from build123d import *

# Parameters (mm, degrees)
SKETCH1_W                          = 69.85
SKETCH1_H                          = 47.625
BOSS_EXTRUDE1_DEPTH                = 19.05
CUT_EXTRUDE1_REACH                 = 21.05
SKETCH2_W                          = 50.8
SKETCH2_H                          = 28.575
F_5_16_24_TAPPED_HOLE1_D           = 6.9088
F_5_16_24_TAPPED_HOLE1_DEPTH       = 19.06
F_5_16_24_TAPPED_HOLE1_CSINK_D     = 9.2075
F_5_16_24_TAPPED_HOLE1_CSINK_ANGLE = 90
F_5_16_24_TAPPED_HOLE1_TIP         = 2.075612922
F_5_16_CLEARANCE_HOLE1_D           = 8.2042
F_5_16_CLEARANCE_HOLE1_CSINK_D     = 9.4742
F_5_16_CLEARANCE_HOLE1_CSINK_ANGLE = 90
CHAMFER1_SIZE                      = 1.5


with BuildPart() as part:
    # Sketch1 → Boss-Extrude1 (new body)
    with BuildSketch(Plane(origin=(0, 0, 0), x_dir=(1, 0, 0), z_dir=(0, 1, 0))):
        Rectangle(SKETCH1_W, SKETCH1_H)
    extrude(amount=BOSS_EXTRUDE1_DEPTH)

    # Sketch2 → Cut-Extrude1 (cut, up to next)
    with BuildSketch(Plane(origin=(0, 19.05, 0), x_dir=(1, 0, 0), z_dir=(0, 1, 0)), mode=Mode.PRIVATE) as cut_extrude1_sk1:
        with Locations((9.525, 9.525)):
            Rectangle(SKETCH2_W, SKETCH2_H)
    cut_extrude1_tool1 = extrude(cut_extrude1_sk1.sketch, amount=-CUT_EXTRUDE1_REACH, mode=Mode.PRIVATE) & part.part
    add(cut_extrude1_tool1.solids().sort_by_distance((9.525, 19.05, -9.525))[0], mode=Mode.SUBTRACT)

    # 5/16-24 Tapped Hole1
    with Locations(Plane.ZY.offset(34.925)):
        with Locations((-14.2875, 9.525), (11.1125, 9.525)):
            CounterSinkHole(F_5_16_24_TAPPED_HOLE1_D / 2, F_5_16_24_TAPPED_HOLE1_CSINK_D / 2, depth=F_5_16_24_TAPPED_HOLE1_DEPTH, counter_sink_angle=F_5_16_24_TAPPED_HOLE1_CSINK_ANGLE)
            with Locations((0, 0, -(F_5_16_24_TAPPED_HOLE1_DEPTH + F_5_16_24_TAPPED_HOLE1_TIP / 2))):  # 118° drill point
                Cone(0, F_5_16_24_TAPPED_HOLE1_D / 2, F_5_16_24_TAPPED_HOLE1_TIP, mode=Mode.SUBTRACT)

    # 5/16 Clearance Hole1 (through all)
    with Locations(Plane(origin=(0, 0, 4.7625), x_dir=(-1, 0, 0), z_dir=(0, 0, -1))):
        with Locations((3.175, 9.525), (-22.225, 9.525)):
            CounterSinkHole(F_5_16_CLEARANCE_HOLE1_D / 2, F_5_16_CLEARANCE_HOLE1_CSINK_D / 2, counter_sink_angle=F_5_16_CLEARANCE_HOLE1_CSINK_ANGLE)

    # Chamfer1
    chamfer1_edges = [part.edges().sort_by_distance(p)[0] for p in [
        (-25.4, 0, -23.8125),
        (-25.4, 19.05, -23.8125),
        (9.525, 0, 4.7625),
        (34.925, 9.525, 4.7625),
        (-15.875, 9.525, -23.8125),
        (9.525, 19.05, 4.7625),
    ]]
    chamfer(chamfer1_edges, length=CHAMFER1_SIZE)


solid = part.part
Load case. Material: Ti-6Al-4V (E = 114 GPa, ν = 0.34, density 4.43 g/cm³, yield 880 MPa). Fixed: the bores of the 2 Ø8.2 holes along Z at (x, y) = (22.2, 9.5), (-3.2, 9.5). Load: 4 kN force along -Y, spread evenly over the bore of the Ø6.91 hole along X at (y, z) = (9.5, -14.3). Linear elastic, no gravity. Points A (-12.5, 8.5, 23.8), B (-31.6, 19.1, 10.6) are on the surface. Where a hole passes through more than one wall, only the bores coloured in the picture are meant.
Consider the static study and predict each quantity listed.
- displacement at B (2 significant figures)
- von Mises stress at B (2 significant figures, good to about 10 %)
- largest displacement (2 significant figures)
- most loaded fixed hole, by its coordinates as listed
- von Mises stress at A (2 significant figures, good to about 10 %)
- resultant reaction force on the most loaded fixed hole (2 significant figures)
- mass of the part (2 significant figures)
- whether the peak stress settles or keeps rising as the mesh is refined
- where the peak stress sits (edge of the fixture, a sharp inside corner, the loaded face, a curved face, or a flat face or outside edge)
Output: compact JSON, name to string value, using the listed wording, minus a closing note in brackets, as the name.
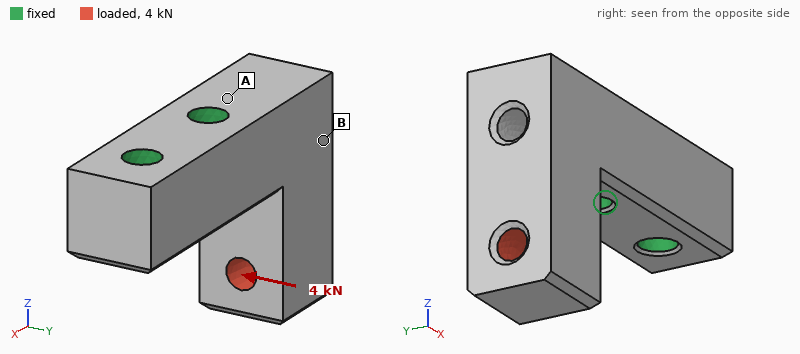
{"displacement at B": "0.041 mm", "von Mises stress at B": "34 MPa", "largest displacement": "0.15 mm", "most loaded fixed hole, by its coordinates as listed": "(-3.2, 9.5)", "von Mises stress at A": "76 MPa", "resultant reaction force on the most loaded fixed hole": "4.9 kN", "mass of the part": "140 g", "whether the peak stress settles or keeps rising as the mesh is refined": "keeps rising", "where the peak stress sits": "edge of the fixture"}
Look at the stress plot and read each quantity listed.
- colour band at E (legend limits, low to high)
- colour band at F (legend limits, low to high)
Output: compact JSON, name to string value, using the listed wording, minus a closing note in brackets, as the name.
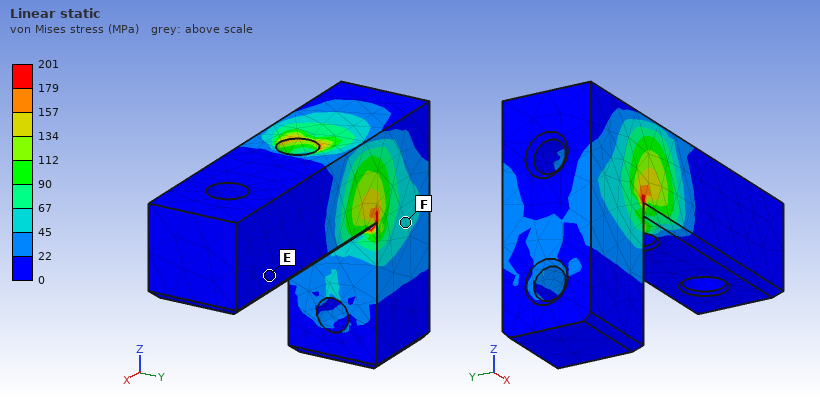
{"colour band at E": "0 to 22 MPa", "colour band at F": "45 to 67 MPa"}
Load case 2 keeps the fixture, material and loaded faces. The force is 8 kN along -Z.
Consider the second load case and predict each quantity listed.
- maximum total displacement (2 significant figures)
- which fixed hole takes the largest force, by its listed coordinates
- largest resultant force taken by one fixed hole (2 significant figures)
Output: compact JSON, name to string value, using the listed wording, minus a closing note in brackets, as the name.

{"maximum total displacement": "81 µm", "which fixed hole takes the largest force, by its listed coordinates": "(-3.2, 9.5)", "largest resultant force taken by one fixed hole": "8.4 kN"}
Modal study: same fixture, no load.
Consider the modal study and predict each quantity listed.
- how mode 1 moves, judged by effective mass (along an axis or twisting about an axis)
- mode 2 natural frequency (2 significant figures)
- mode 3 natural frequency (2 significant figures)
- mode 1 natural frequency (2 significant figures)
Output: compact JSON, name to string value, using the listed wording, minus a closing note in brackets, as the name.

{"how mode 1 moves, judged by effective mass": "along Y", "mode 2 natural frequency": "5600 Hz", "mode 3 natural frequency": "11 kHz", "mode 1 natural frequency": "5200 Hz"}
